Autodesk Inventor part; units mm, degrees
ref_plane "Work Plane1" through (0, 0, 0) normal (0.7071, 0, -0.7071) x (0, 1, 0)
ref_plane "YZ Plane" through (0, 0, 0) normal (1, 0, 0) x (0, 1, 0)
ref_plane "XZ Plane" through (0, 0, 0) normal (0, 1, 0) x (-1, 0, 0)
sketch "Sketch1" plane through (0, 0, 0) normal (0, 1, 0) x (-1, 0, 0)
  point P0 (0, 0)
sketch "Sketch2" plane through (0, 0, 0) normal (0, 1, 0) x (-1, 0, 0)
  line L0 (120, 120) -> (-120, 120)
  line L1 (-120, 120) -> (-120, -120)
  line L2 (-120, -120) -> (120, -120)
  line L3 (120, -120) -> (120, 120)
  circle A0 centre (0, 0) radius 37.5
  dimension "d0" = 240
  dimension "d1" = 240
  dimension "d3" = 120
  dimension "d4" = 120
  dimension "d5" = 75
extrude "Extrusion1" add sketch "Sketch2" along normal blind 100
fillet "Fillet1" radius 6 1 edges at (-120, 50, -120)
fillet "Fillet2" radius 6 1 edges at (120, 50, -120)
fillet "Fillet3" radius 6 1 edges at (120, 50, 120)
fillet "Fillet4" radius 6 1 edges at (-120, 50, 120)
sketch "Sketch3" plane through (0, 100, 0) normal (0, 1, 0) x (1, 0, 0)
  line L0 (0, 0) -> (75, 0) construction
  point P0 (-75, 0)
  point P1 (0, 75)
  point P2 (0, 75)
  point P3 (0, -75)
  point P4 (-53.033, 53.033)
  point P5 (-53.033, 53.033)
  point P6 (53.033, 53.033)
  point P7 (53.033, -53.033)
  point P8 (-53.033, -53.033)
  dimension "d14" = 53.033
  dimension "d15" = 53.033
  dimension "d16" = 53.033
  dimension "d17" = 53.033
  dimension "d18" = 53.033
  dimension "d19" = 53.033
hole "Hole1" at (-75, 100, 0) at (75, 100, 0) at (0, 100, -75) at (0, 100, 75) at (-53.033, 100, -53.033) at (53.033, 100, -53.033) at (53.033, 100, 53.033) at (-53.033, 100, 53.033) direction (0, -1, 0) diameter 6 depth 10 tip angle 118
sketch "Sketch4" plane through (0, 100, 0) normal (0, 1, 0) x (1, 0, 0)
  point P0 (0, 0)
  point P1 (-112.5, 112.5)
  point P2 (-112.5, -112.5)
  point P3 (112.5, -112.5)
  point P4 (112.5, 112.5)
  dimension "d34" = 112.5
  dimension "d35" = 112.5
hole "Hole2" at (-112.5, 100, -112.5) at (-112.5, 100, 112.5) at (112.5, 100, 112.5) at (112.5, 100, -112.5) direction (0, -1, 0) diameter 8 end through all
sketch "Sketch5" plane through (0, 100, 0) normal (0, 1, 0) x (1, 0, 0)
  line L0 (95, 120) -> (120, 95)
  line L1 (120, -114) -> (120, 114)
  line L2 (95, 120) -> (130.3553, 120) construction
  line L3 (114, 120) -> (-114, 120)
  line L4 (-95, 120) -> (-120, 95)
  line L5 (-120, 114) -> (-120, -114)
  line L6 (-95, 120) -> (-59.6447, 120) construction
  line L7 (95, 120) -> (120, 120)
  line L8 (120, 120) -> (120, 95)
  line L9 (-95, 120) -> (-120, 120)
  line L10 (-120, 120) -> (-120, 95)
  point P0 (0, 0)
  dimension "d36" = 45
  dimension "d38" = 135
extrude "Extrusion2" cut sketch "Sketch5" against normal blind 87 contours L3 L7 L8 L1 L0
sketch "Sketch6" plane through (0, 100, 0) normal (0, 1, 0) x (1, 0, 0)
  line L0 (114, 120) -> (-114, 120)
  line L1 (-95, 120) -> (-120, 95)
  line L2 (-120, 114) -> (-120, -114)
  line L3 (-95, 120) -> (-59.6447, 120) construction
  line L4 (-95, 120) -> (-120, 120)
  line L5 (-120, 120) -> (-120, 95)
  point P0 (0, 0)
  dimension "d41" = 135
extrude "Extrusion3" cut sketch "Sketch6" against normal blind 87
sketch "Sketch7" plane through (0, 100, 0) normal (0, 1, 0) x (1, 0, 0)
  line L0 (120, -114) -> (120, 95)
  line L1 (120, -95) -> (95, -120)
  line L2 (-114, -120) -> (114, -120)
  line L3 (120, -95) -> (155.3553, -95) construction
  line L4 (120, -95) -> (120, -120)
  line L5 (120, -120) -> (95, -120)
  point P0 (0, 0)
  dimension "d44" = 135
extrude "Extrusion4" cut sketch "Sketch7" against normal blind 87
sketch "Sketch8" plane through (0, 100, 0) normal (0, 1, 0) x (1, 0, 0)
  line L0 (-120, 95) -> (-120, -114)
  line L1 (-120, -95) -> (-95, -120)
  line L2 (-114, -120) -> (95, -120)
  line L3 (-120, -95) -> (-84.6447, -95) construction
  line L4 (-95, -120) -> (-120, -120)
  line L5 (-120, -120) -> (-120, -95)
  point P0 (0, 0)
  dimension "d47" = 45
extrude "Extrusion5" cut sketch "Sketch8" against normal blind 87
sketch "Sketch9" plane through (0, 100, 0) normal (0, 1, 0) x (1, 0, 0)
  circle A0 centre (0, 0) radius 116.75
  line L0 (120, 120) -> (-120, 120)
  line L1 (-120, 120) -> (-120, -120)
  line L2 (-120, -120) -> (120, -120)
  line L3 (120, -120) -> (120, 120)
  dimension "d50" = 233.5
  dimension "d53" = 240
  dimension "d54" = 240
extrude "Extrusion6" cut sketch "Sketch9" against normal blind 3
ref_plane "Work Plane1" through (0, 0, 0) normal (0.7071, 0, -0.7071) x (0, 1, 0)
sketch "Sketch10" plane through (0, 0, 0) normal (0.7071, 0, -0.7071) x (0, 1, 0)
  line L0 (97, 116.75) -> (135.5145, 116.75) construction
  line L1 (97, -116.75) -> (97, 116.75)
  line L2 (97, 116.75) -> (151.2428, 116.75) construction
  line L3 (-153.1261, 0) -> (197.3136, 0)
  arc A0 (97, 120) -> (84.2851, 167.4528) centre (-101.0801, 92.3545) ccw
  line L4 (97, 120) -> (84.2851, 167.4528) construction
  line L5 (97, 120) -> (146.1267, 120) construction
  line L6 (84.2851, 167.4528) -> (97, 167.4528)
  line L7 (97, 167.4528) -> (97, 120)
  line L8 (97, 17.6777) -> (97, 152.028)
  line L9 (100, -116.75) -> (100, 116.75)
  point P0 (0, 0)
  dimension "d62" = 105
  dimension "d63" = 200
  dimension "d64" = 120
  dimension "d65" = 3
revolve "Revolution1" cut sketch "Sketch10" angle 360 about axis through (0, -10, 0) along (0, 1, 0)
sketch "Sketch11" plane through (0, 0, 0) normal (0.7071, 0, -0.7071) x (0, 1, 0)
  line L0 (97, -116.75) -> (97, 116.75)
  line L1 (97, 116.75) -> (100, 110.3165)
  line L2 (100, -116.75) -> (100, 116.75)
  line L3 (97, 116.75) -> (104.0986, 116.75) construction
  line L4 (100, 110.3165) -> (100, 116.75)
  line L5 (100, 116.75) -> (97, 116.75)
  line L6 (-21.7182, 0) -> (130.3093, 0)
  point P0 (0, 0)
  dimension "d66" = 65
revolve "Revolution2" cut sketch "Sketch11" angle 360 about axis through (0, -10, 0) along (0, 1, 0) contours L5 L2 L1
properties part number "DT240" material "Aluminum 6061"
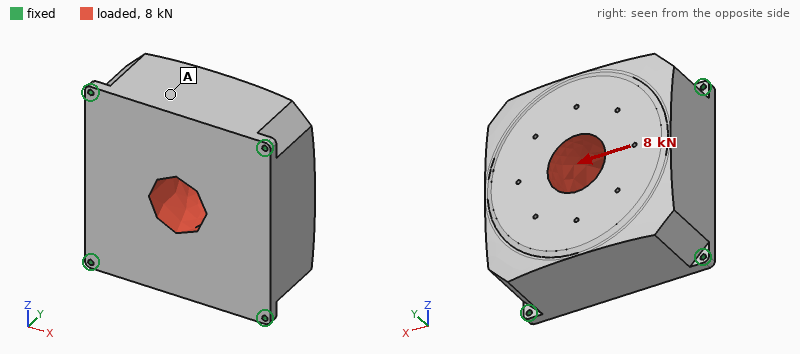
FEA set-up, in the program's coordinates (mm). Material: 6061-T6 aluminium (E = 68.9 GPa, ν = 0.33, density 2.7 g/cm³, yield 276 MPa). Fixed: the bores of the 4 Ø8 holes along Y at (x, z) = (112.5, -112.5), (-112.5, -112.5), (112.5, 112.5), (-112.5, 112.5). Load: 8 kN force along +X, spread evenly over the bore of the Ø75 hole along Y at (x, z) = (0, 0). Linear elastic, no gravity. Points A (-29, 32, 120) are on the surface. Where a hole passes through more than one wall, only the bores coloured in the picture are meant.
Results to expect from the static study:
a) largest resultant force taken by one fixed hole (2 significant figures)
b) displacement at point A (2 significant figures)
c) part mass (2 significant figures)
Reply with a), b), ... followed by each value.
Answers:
a) 2.3 kN
b) 3.0 µm
c) 14 kg
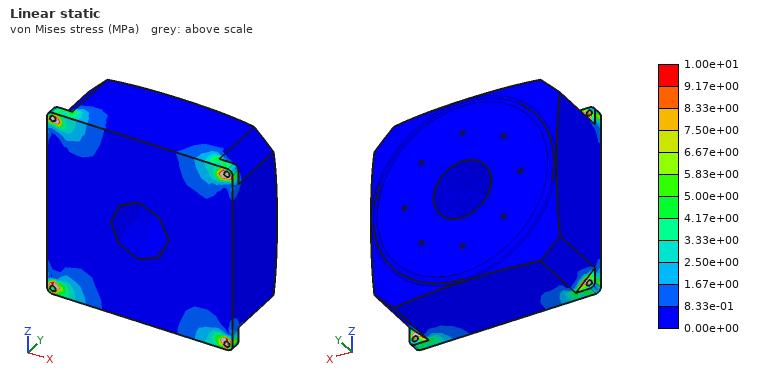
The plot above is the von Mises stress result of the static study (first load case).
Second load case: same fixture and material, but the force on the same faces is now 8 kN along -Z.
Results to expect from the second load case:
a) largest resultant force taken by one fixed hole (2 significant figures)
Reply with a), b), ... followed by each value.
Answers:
a) 2.3 kN
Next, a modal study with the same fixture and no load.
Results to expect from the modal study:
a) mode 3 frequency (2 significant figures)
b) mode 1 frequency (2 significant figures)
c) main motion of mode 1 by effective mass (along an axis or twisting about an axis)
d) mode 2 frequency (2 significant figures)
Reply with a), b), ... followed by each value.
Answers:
a) 2000 Hz
b) 1700 Hz
c) along Y
d) 2000 Hz
